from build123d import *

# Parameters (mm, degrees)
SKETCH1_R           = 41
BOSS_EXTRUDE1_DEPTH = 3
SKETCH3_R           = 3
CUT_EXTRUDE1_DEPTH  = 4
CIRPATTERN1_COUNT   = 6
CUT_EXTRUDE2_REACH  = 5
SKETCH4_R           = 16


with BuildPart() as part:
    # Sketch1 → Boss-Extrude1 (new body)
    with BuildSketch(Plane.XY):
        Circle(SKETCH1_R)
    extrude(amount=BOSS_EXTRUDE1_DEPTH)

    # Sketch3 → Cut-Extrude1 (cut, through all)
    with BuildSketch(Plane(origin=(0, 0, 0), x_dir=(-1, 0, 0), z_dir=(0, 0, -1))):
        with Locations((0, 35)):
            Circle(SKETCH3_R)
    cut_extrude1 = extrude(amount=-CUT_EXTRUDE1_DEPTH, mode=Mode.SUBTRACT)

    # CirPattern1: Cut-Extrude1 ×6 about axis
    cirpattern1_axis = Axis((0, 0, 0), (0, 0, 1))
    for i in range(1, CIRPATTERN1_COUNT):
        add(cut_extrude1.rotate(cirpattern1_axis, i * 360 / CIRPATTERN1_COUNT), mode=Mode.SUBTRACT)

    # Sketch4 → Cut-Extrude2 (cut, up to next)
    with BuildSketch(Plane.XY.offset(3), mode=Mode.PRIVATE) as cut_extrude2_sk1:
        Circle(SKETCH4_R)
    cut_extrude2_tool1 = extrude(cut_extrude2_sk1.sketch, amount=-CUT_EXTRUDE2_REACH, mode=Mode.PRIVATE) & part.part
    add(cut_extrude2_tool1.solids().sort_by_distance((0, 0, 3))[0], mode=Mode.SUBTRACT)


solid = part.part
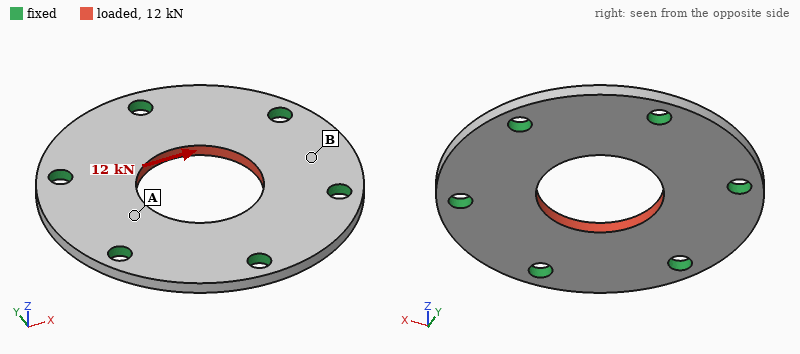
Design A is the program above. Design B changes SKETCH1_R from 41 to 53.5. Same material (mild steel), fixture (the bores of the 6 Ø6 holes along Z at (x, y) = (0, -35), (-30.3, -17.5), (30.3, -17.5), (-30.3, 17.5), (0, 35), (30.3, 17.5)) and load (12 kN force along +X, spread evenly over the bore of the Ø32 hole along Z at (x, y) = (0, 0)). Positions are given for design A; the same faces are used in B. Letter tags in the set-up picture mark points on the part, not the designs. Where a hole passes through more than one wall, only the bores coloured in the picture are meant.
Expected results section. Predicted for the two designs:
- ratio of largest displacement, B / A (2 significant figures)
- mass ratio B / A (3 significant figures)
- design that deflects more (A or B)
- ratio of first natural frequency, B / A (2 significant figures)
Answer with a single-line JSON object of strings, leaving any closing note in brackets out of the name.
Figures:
{"ratio of largest displacement, B / A": "0.92", "mass ratio B / A": "1.86", "design that deflects more": "A", "ratio of first natural frequency, B / A": "0.65"}
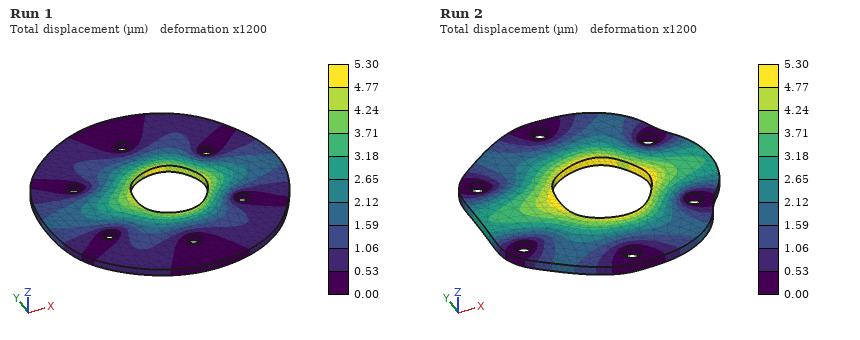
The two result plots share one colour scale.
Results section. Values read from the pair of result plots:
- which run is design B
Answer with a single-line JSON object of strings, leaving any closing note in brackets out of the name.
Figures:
{"which run is design B": "Run 1"}
